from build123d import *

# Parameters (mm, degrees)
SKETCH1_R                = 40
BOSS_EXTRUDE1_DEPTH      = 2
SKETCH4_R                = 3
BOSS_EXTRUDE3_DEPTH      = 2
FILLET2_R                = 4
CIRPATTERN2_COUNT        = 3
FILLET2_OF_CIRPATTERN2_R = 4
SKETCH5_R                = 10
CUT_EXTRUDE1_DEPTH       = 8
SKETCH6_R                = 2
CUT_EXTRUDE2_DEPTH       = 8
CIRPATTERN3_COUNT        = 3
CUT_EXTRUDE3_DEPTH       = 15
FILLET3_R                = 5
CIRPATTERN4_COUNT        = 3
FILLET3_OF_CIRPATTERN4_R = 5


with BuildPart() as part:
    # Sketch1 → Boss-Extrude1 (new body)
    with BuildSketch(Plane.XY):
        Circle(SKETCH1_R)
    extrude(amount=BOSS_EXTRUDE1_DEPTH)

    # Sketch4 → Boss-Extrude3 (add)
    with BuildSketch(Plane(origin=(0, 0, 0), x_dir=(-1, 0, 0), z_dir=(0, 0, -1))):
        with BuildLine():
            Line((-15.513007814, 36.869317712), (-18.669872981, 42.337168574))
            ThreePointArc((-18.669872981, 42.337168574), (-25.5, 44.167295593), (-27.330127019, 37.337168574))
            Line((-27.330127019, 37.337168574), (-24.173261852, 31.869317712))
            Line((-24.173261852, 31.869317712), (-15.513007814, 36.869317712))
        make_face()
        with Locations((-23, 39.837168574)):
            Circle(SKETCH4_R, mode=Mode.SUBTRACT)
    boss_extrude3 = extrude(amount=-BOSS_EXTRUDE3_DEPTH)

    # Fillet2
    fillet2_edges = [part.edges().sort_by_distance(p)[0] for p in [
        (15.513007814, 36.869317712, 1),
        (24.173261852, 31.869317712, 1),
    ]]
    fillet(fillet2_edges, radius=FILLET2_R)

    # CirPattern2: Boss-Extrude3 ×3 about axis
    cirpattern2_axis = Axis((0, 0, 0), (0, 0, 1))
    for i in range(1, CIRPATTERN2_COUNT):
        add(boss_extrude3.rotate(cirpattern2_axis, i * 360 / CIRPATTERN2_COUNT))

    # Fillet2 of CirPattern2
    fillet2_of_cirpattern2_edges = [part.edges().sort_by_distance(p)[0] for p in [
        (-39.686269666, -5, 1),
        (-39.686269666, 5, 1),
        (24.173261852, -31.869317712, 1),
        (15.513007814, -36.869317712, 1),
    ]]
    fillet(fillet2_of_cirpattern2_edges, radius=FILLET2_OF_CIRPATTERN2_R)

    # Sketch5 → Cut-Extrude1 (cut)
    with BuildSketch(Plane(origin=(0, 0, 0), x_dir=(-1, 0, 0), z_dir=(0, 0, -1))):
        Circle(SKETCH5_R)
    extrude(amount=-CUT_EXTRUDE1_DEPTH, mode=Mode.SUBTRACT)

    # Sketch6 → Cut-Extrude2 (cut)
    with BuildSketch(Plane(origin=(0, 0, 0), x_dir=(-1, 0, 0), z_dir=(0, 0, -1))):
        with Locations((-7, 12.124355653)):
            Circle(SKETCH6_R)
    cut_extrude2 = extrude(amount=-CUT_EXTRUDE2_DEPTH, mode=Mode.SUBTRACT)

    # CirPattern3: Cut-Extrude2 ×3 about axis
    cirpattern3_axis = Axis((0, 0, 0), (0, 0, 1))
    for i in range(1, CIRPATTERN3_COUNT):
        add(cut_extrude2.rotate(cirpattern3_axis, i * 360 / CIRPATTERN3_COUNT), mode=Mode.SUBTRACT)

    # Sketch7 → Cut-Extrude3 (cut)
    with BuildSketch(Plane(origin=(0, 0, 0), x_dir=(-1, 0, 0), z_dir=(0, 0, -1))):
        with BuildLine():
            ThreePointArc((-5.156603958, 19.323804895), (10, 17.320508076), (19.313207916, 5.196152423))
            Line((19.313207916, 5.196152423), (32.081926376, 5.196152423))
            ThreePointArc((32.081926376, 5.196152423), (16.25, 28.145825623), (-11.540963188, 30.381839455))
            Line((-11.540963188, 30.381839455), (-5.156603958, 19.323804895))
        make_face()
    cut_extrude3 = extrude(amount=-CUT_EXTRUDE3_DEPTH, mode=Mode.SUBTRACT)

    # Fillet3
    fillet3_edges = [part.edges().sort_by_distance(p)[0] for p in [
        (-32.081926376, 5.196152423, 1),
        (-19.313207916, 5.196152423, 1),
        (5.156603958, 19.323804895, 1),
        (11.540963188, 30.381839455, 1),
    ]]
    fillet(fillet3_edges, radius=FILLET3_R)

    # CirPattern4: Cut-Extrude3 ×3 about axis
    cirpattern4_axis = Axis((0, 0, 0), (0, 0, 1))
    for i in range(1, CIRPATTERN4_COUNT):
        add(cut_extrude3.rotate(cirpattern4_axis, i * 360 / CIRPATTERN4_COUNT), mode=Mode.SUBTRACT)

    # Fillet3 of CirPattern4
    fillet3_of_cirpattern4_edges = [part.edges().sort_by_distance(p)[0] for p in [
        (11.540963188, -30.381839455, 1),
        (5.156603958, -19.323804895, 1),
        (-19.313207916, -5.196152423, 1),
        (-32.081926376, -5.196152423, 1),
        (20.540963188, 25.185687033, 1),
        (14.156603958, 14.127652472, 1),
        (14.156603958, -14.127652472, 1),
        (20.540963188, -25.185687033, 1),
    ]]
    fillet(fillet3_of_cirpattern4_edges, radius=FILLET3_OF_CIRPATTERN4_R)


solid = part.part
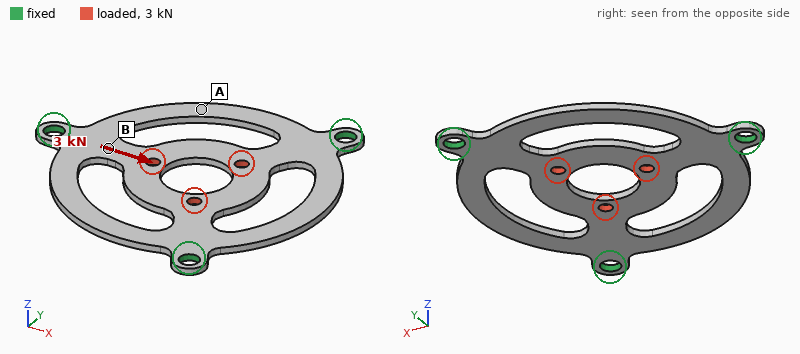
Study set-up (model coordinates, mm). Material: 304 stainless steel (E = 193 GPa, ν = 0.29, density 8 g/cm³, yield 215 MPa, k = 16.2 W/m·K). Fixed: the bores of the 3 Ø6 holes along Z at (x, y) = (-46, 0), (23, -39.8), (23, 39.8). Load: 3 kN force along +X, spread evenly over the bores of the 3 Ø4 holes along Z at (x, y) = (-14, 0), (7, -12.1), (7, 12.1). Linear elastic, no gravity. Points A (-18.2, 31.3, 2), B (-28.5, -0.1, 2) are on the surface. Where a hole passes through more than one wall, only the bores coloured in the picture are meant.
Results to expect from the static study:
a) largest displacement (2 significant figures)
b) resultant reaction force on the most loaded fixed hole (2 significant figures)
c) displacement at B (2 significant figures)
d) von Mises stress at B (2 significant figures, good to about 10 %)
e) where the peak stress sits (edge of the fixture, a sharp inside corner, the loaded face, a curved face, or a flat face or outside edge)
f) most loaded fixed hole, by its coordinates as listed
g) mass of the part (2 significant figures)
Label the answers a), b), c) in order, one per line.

a) 26 µm
b) 1.6 kN
c) 5.8 µm
d) 67 MPa
e) a curved face
f) (-46, 0)
g) 53 g
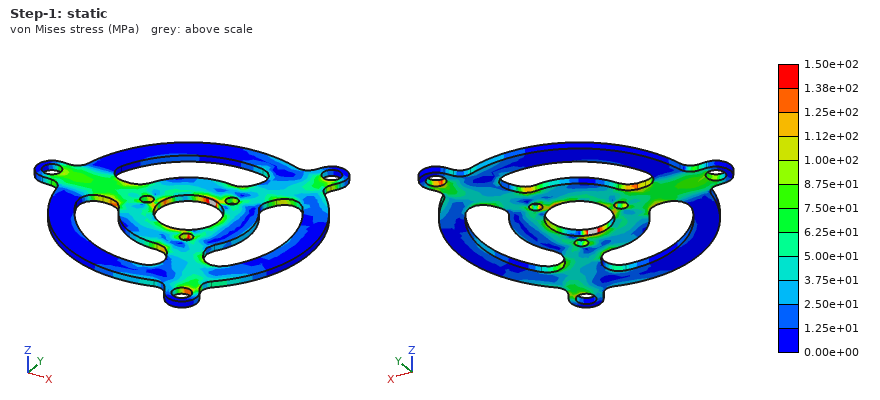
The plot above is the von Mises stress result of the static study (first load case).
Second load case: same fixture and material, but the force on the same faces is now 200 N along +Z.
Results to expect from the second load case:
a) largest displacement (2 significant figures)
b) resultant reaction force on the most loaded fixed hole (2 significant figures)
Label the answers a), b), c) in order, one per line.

a) 0.15 mm
b) 67 N
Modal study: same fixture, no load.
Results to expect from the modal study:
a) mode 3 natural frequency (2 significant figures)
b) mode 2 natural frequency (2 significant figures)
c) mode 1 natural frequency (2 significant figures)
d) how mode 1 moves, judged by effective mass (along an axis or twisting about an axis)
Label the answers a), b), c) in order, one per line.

a) 1500 Hz
b) 1500 Hz
c) 1400 Hz
d) along Z
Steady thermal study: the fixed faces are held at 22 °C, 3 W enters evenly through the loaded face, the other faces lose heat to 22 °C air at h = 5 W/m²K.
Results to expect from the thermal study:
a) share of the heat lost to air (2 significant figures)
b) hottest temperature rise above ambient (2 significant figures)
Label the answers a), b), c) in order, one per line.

a) 33 %
b) 60 K
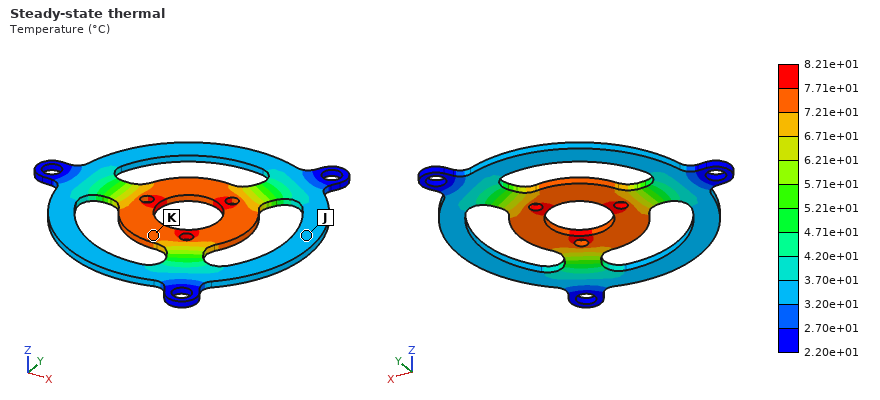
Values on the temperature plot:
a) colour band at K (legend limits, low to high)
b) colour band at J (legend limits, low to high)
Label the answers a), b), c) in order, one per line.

a) 7.21e+01 to 7.71e+01 °C
b) 3.20e+01 to 3.70e+01 °C
